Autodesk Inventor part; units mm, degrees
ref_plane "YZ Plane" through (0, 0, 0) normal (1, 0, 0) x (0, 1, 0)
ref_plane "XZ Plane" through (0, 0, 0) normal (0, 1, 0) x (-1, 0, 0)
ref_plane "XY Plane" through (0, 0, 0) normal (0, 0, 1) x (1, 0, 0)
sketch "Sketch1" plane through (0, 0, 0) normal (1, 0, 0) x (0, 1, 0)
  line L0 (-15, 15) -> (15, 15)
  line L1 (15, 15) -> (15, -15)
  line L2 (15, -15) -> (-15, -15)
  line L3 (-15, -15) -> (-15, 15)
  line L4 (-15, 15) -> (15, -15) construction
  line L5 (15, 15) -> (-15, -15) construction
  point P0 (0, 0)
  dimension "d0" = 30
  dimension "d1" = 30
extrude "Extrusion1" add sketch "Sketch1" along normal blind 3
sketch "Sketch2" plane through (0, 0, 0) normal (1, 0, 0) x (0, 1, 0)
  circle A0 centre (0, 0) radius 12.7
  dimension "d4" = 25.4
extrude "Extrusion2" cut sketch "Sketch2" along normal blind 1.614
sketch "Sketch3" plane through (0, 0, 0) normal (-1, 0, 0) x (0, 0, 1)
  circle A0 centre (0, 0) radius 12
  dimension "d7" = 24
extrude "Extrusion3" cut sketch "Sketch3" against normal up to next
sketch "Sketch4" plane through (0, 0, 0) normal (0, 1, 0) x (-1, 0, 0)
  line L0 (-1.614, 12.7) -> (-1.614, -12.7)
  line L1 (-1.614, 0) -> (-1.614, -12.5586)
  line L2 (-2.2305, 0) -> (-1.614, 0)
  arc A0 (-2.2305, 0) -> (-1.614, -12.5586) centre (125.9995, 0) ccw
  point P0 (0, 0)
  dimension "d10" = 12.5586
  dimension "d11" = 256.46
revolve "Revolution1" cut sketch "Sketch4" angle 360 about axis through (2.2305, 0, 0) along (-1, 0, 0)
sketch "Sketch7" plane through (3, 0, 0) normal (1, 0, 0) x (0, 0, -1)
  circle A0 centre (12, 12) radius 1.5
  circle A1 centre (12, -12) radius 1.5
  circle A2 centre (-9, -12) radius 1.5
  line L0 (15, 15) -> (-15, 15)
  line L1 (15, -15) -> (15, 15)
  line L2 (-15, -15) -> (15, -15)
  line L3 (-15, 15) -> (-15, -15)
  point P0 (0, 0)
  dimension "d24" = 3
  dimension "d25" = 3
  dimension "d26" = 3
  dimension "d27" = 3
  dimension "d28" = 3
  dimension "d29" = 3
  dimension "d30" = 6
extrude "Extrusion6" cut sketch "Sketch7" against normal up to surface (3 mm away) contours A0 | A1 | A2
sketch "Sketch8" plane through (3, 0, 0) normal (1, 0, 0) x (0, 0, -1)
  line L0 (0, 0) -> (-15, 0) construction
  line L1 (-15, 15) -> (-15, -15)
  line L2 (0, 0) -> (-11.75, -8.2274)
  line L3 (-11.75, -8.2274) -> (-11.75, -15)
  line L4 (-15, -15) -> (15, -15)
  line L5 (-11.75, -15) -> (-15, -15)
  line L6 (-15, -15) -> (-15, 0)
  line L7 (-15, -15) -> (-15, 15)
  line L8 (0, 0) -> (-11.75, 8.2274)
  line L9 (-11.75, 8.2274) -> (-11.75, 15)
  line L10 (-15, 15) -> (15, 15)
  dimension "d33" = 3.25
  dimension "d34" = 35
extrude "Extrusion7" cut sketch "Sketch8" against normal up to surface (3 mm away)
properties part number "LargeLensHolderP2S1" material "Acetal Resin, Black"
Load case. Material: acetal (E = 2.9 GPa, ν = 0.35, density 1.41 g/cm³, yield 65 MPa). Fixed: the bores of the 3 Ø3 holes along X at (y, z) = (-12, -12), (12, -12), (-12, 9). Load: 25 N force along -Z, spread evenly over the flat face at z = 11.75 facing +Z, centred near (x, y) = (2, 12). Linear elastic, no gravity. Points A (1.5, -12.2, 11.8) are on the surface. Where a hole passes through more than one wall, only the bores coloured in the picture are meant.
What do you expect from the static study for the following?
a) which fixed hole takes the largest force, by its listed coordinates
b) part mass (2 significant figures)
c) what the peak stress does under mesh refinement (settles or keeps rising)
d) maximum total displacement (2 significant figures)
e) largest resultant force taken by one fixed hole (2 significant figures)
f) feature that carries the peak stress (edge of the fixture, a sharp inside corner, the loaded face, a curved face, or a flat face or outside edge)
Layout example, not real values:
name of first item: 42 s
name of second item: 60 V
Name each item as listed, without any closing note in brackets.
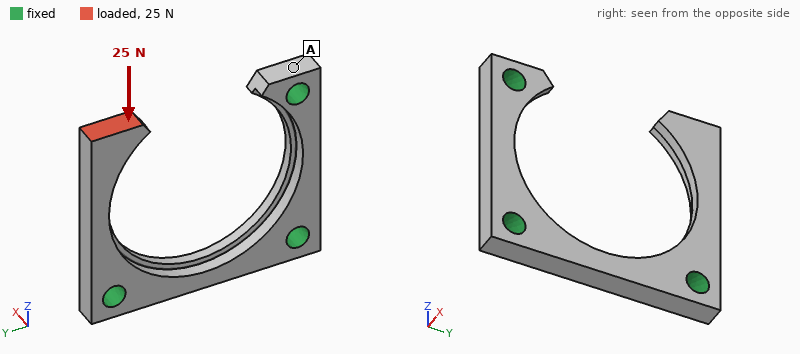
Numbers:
which fixed hole takes the largest force, by its listed coordinates: (12, -12)
part mass: 1.3 g
what the peak stress does under mesh refinement: keeps rising
maximum total displacement: 0.42 mm
largest resultant force taken by one fixed hole: 25 N
feature that carries the peak stress: a sharp inside corner
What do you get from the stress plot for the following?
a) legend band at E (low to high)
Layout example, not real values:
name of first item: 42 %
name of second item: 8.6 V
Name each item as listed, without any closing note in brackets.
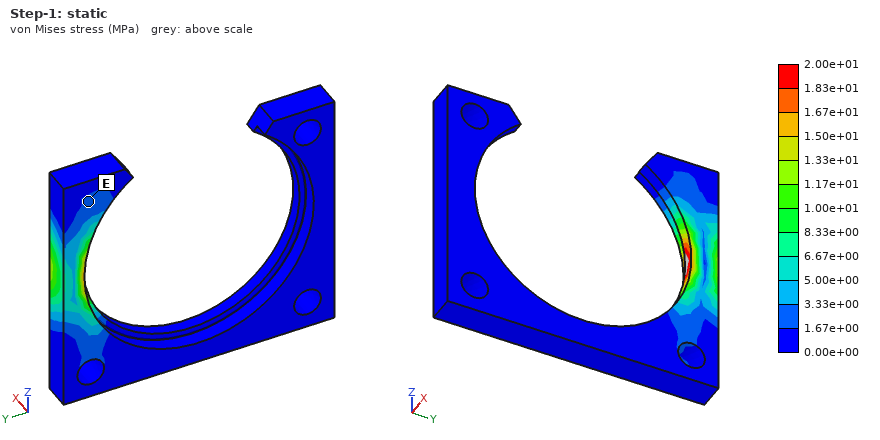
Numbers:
legend band at E: 1.67e+00 to 3.33e+00 MPa
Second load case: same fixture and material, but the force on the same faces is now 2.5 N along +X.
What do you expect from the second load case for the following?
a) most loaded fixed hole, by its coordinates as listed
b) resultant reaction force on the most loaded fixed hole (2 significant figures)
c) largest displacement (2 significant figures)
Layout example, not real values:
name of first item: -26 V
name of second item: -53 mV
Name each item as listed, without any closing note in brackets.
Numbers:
most loaded fixed hole, by its coordinates as listed: (12, -12)
resultant reaction force on the most loaded fixed hole: 2.7 N
largest displacement: 0.44 mm
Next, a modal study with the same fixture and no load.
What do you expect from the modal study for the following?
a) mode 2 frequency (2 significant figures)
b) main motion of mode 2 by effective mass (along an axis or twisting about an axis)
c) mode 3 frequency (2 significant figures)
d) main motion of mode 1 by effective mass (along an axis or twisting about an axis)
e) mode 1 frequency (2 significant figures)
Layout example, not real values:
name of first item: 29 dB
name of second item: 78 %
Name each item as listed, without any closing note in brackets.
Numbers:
mode 2 frequency: 1400 Hz
main motion of mode 2 by effective mass: along Y
mode 3 frequency: 4800 Hz
main motion of mode 1 by effective mass: along X
mode 1 frequency: 1100 Hz
